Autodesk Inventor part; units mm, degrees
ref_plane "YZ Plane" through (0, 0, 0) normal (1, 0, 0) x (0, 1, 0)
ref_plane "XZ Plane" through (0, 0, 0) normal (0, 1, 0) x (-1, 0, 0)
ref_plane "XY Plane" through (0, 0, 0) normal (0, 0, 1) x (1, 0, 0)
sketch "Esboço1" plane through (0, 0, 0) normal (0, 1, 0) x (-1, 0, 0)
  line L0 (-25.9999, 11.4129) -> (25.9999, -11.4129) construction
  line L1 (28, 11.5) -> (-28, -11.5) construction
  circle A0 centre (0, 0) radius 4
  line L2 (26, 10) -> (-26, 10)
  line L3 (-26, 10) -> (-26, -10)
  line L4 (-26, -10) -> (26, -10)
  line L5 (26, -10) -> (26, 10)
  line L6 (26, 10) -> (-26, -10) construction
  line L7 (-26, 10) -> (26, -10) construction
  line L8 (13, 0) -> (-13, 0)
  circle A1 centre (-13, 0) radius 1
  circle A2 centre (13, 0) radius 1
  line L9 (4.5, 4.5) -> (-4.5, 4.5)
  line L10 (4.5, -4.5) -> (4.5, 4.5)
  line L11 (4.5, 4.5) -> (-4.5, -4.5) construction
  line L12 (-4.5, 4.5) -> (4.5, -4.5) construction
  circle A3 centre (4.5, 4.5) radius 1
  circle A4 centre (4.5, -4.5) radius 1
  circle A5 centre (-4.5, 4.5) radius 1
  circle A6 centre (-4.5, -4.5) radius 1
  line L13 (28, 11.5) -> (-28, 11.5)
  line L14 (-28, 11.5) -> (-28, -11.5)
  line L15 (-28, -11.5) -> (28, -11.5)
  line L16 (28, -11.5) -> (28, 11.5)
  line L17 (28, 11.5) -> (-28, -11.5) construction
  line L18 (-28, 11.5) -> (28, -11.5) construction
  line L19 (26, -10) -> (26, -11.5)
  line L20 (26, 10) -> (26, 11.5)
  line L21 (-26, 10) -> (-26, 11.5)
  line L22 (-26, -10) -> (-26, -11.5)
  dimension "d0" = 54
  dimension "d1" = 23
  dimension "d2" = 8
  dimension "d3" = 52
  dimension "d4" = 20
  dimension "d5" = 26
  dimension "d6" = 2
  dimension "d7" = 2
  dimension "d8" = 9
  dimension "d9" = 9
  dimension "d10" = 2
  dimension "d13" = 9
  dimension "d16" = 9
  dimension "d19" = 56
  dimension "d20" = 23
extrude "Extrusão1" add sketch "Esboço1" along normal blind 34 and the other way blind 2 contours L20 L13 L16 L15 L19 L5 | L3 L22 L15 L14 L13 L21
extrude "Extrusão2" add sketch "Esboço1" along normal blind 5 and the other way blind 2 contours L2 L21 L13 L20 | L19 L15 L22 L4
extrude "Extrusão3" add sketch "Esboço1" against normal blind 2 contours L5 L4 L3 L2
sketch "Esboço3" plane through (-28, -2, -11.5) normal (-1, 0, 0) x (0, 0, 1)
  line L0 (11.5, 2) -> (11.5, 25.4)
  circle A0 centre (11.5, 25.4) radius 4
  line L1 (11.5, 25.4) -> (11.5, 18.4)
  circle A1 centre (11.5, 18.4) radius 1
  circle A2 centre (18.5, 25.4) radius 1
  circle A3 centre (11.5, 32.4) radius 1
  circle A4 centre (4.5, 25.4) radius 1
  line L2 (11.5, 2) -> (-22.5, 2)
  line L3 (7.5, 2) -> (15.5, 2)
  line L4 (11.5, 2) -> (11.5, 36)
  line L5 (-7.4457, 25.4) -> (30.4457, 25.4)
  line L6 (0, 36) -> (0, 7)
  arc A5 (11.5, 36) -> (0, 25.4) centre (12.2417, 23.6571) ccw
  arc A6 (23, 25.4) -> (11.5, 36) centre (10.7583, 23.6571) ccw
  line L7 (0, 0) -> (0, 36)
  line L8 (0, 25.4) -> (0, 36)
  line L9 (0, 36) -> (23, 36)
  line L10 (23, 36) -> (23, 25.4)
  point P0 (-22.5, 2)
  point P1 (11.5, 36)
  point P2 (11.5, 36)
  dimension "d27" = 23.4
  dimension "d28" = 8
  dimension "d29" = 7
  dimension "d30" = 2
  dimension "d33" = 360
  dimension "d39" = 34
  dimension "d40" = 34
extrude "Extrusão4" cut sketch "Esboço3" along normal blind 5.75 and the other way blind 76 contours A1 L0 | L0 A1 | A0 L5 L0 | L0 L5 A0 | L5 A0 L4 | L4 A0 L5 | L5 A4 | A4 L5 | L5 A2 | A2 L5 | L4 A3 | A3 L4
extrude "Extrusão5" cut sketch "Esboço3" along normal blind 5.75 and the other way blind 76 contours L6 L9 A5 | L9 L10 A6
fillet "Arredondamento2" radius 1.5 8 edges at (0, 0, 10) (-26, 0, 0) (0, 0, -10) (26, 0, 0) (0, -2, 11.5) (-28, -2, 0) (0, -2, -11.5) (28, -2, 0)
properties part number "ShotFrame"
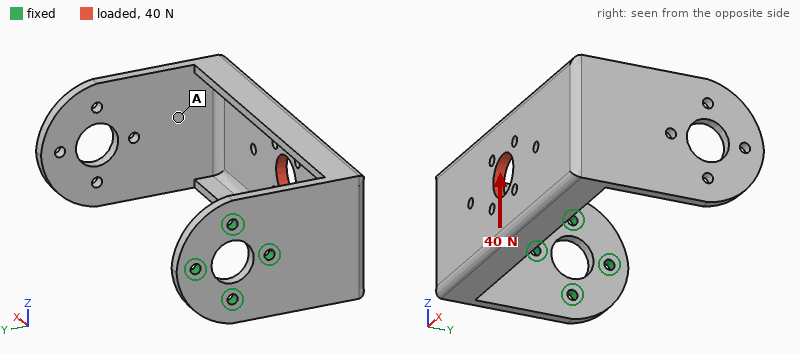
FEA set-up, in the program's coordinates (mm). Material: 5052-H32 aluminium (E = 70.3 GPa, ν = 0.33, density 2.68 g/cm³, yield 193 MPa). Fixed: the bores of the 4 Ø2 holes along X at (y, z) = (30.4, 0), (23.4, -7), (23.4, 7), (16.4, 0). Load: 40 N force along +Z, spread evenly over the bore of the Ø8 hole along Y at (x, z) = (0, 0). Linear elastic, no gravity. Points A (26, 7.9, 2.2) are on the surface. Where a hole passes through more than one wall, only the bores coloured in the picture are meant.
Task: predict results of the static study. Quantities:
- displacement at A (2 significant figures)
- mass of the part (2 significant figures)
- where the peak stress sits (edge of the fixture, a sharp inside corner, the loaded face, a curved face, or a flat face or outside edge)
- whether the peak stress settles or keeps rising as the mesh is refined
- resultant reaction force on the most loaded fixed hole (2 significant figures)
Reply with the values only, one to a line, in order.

0.42 mm
16 g
edge of the fixture
keeps rising
49 N
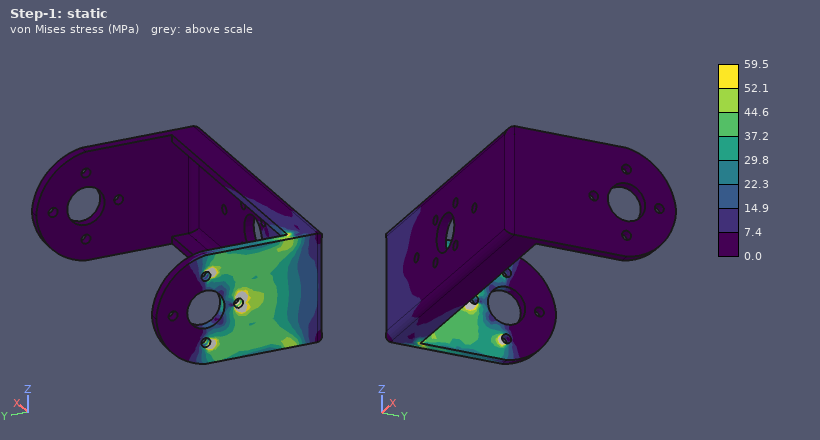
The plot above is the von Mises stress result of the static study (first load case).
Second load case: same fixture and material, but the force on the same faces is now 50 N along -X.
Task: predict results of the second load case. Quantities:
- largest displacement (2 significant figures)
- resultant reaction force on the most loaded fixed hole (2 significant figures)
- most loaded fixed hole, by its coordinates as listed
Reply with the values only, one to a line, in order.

0.42 mm
100 N
(16.4, 0)
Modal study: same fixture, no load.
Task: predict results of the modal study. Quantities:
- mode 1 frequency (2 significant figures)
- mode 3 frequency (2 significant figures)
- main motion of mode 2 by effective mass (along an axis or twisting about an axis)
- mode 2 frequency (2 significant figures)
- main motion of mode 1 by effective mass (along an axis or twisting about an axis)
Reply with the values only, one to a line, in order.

290 Hz
1300 Hz
along Z
390 Hz
along Y
